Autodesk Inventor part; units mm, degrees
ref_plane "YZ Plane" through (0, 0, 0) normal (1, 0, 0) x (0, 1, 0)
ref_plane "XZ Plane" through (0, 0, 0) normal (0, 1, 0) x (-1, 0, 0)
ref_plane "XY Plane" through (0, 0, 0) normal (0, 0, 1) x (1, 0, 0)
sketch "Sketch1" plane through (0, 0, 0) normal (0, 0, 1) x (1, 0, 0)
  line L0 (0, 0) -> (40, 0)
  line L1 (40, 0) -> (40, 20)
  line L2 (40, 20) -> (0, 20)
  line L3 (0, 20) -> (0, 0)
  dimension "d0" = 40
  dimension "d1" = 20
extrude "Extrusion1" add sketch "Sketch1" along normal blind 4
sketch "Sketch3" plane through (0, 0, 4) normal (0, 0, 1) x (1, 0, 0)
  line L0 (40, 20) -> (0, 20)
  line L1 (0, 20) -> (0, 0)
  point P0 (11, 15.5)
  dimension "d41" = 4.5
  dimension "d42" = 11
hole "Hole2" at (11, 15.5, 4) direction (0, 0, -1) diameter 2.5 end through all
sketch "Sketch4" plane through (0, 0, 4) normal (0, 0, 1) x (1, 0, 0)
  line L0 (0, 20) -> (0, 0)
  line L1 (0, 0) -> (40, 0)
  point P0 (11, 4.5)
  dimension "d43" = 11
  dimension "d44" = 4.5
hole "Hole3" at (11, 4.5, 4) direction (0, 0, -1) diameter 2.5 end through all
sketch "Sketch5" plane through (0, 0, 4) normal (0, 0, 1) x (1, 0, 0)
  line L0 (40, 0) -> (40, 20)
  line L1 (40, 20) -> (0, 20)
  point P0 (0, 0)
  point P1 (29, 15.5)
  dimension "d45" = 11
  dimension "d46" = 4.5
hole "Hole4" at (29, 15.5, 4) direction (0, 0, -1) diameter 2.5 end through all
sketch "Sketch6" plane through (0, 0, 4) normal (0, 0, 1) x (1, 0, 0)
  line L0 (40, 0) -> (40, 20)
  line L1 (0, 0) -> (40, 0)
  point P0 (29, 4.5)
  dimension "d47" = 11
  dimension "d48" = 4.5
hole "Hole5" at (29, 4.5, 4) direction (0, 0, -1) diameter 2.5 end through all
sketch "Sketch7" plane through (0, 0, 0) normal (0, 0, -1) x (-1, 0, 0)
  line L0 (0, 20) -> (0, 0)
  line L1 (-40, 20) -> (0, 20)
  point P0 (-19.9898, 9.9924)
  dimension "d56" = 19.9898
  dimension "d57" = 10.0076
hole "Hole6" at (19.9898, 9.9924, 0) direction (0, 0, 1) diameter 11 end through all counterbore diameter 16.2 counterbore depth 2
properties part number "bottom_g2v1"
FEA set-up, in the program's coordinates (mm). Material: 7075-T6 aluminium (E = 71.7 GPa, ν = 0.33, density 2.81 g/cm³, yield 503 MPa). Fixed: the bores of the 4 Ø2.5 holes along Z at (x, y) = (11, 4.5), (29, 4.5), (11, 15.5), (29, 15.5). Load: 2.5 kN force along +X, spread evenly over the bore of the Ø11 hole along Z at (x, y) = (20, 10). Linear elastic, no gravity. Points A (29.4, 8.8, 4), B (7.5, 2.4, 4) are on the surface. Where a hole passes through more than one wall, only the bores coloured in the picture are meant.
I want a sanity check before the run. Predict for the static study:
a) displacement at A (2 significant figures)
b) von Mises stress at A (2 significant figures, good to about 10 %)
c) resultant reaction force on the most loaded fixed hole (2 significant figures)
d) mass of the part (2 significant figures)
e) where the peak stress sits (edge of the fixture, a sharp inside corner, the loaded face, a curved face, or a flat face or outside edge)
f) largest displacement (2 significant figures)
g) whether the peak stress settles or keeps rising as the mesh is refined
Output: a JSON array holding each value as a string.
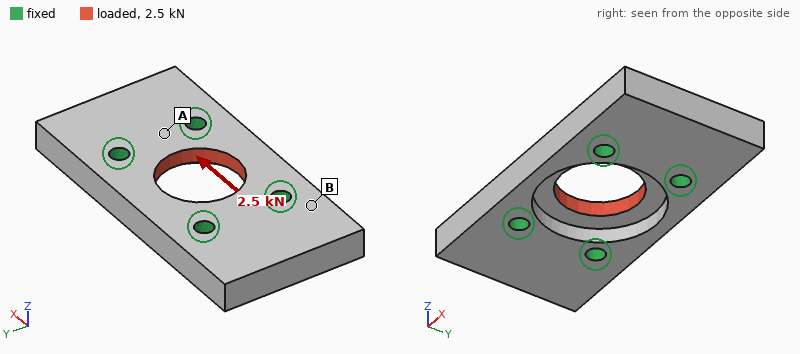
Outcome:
["1.7 µm", "22 MPa", "640 N", "7.1 g", "edge of the fixture", "4.0 µm", "keeps rising"]
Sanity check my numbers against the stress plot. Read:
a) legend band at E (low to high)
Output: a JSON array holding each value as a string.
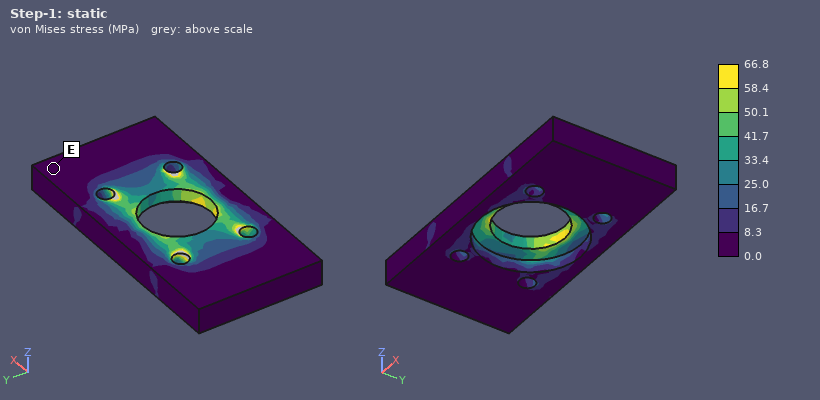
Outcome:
["0.0 to 8.3 MPa"]
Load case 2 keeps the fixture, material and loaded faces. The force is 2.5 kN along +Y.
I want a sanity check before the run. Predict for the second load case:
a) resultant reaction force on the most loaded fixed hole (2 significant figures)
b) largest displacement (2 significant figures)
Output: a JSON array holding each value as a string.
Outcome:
["640 N", "11 µm"]
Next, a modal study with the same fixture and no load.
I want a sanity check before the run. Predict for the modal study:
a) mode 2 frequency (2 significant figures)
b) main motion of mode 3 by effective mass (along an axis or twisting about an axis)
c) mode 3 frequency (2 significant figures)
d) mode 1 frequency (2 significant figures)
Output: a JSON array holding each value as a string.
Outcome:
["24 kHz", "twisting about X", "36 kHz", "24 kHz"]
